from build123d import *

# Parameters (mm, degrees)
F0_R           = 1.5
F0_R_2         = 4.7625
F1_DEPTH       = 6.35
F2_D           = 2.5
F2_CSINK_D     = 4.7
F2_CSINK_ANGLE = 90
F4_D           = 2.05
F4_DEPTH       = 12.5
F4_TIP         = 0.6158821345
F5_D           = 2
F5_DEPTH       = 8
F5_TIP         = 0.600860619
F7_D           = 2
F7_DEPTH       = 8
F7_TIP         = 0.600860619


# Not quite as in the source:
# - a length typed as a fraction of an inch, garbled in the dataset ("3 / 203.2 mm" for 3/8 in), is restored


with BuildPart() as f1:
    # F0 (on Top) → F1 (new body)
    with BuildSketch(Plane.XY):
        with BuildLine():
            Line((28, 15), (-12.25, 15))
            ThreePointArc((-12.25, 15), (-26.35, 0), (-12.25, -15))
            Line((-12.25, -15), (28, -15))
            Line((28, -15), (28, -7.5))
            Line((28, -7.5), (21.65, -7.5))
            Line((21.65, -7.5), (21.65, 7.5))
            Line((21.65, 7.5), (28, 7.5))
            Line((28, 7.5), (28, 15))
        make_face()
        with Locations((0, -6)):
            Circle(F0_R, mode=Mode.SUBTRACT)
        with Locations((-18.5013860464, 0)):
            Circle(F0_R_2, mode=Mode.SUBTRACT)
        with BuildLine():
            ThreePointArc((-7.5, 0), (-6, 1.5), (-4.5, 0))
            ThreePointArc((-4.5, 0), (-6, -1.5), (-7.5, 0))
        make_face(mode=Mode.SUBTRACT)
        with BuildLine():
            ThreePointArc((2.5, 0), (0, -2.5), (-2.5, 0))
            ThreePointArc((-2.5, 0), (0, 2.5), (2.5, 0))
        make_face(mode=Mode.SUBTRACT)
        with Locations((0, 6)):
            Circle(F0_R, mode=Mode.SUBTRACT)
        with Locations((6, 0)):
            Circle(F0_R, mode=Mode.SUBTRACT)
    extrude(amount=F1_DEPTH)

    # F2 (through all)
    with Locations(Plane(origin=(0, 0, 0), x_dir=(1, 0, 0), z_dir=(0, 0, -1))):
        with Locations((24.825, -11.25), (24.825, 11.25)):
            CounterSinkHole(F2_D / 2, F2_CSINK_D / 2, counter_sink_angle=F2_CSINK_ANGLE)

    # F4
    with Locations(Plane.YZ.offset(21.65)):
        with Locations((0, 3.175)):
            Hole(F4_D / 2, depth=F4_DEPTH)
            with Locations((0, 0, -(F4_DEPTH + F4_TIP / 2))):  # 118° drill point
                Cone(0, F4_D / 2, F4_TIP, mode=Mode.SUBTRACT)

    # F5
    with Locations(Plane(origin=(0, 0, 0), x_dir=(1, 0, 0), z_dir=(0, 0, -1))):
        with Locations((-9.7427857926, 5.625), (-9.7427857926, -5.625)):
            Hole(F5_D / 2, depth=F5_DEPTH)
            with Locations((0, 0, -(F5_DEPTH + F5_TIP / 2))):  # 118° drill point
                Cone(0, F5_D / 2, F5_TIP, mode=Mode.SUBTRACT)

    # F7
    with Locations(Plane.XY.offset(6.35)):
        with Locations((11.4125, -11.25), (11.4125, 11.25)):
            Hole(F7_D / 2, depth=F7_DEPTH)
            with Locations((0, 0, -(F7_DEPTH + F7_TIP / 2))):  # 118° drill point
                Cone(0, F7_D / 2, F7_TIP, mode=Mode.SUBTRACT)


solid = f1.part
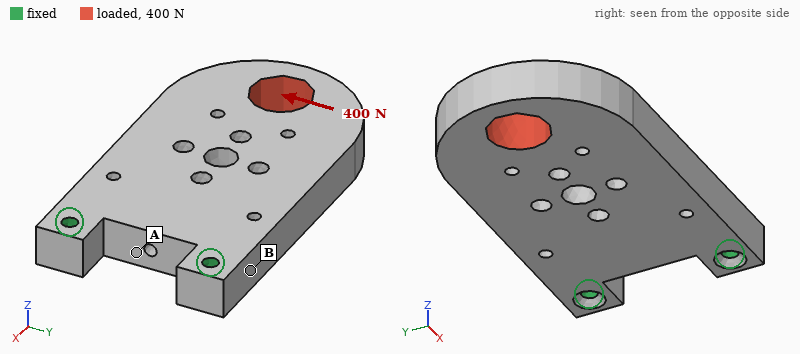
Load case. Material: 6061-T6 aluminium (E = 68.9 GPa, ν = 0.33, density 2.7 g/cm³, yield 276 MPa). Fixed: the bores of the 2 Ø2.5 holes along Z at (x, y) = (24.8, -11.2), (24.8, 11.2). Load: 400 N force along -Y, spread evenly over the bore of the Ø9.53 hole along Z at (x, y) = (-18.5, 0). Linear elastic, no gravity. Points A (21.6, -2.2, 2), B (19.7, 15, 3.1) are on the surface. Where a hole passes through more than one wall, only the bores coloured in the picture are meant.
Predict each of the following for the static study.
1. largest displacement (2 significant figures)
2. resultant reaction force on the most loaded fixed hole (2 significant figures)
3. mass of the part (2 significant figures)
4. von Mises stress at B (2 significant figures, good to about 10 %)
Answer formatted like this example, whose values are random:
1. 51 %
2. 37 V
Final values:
1. 23 µm
2. 750 N
3. 22 g
4. 13 MPa
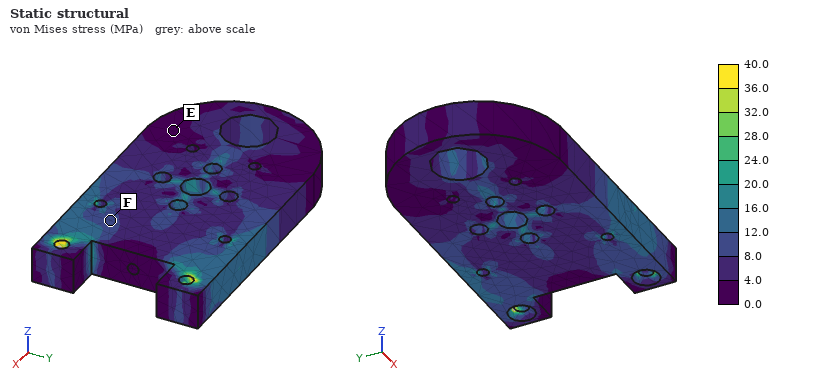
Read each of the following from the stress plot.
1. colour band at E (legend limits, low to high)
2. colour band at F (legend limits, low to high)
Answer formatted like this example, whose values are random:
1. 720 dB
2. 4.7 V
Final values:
1. 0.0 to 4.0 MPa
2. 8.0 to 12.0 MPa
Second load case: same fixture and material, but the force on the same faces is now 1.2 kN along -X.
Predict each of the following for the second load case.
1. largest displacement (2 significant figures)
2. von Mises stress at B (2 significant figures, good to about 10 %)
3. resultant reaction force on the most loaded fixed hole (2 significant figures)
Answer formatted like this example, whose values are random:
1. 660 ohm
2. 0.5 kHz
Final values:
1. 9.5 µm
2. 8.4 MPa
3. 610 N
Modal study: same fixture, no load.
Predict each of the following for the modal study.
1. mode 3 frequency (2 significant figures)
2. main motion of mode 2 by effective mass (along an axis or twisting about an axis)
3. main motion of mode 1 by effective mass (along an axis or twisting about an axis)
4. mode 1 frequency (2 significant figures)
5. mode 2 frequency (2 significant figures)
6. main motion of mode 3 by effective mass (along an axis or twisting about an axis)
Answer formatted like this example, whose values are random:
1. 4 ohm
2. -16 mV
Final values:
1. 8000 Hz
2. twisting about X
3. along Z
4. 1900 Hz
5. 7000 Hz
6. along Y
